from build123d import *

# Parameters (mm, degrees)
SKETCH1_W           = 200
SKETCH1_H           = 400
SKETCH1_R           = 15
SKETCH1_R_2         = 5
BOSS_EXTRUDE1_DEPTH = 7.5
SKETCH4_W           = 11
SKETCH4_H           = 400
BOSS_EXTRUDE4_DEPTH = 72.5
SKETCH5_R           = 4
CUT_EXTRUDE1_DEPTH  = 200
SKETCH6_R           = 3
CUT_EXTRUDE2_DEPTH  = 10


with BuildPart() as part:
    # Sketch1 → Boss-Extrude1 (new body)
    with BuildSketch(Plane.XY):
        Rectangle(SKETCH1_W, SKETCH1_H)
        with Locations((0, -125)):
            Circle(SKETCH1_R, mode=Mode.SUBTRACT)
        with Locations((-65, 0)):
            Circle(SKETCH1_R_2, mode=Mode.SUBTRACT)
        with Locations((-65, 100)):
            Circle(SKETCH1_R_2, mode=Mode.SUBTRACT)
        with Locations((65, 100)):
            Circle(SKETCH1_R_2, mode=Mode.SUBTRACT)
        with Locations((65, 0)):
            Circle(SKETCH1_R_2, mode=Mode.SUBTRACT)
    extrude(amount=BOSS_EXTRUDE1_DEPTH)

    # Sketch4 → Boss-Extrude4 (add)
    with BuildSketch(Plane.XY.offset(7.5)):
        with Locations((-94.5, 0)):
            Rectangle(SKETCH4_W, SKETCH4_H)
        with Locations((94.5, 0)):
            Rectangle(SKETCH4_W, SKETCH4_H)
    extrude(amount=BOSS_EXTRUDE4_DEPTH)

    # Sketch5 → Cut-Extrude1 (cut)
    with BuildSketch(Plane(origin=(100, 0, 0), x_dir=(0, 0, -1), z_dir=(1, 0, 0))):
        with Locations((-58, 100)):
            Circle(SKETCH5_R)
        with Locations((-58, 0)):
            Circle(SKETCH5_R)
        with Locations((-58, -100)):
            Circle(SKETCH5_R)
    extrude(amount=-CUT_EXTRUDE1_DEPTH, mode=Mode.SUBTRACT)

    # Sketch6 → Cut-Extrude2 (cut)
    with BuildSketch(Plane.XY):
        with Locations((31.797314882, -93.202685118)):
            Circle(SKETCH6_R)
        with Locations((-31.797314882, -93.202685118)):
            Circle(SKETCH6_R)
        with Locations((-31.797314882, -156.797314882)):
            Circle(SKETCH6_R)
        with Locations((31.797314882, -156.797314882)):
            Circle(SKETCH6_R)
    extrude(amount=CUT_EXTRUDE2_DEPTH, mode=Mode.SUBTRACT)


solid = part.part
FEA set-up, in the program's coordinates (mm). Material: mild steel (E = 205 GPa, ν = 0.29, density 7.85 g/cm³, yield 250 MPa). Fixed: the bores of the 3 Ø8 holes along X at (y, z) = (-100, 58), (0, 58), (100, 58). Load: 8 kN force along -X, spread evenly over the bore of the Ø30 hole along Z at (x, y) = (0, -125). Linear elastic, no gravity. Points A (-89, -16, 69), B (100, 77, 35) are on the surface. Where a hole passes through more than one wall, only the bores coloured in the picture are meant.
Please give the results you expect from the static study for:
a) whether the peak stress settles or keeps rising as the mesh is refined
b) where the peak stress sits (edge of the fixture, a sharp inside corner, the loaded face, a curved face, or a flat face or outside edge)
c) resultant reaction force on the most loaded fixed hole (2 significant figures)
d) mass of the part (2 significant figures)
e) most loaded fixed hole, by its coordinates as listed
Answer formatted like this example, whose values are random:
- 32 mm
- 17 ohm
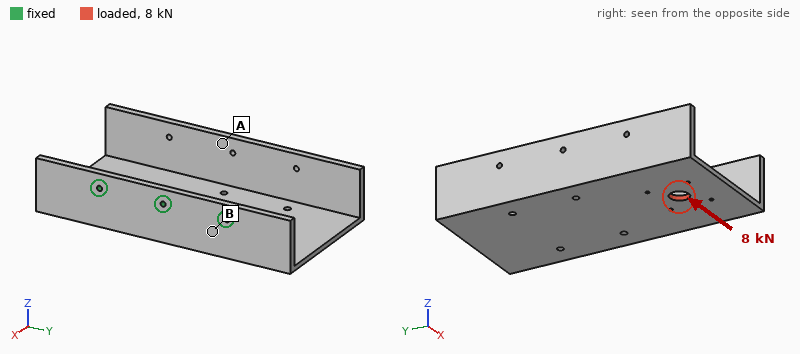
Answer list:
- keeps rising
- edge of the fixture
- 7.3 kN
- 9.6 kg
- (-100, 58)
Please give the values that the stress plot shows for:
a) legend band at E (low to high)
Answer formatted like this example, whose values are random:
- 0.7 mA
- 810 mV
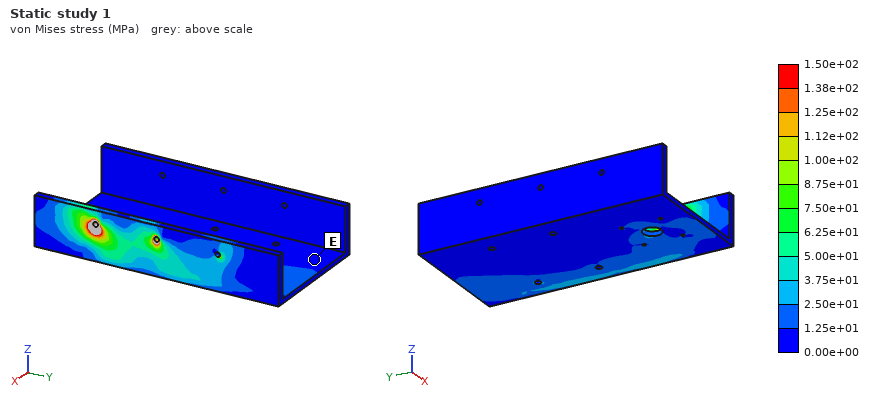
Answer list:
- 0.00e+00 to 1.25e+01 MPa
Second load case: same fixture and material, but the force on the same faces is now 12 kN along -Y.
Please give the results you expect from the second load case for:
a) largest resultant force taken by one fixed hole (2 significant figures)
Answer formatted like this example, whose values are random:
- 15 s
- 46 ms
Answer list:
- 7.3 kN
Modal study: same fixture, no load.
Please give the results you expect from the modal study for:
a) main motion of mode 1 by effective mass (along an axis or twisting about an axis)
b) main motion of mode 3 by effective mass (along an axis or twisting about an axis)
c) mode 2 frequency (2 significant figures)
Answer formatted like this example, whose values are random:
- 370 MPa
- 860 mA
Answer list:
- along Z
- along Y
- 150 Hz
